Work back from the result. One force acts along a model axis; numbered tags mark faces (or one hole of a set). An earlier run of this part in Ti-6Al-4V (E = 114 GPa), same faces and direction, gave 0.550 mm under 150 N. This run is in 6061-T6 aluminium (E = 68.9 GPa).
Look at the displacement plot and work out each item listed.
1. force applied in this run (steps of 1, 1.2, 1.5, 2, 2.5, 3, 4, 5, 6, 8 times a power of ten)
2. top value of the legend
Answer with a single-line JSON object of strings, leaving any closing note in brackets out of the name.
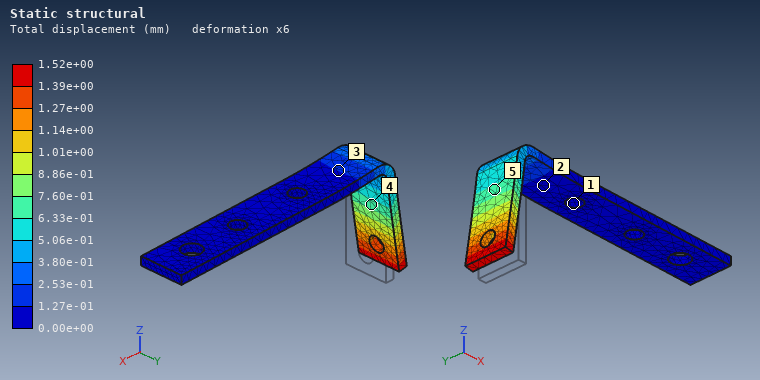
{"force applied in this run": "250 N", "top value of the legend": "1.52e+00 mm"}
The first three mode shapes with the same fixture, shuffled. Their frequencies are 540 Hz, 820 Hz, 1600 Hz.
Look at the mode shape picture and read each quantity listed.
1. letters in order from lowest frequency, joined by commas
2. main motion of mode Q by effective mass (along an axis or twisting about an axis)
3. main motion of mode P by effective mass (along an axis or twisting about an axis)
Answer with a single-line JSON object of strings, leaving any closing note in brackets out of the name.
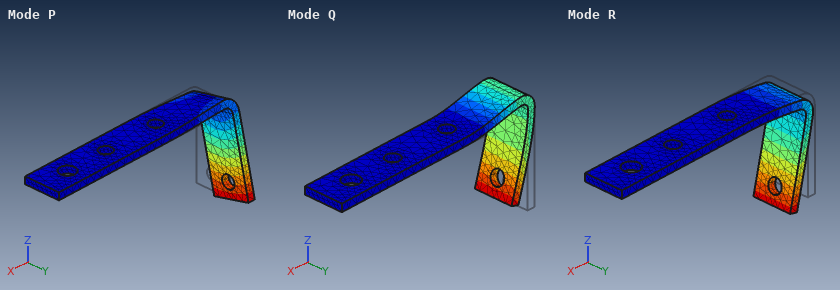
{"letters in order from lowest frequency, joined by commas": "R, P, Q", "main motion of mode Q by effective mass": "along Z", "main motion of mode P by effective mass": "along Y"}
